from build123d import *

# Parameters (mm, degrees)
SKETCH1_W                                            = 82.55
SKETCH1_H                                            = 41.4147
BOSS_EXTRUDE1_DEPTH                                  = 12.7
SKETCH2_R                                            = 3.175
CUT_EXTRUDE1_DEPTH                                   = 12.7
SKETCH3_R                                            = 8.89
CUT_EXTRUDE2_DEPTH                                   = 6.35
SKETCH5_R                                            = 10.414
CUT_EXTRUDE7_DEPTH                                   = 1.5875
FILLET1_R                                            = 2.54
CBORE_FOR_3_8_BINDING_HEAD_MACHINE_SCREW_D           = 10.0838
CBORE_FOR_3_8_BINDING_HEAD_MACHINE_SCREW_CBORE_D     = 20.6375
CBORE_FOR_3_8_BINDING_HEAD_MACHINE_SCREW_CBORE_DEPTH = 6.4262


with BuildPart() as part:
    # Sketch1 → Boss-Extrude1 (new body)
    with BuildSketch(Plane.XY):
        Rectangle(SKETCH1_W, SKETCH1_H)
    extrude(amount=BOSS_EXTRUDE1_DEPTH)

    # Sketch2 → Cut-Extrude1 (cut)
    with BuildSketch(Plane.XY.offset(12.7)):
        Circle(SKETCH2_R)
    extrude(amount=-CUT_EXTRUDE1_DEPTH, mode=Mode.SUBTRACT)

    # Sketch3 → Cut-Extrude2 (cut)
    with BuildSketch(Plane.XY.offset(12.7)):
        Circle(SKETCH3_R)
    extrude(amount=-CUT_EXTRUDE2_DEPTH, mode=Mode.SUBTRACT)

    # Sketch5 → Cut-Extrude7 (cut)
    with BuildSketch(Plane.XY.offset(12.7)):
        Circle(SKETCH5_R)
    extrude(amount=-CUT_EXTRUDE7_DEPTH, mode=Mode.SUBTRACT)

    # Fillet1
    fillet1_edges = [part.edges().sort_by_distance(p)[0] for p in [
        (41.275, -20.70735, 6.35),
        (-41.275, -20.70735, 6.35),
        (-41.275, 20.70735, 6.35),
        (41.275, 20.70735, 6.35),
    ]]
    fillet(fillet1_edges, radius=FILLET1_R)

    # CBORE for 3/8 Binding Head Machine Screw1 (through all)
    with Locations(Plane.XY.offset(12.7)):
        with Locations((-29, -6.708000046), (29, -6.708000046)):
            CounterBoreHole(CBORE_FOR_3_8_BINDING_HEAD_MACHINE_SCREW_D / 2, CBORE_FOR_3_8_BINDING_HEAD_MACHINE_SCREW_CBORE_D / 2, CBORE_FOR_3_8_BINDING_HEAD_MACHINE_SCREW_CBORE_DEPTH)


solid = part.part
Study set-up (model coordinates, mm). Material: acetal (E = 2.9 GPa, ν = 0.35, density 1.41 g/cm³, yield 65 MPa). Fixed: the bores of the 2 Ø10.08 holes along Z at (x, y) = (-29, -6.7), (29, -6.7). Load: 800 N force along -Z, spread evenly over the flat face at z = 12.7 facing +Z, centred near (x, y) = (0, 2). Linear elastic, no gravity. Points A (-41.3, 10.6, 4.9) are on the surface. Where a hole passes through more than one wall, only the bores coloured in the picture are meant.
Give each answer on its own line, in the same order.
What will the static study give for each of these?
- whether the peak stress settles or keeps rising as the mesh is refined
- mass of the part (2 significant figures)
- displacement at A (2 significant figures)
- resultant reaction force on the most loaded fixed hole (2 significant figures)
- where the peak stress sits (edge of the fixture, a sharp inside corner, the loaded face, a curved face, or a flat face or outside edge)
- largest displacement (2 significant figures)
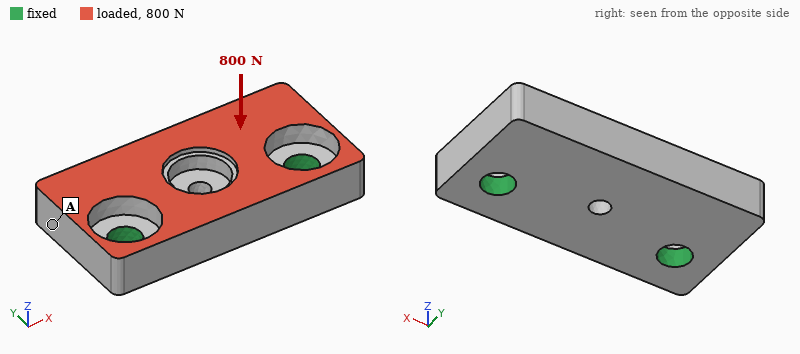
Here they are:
keeps rising
51 g
0.070 mm
410 N
edge of the fixture
0.20 mm
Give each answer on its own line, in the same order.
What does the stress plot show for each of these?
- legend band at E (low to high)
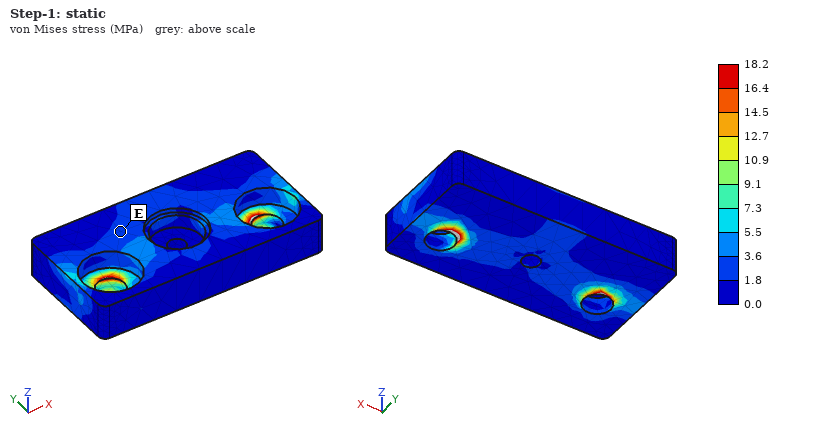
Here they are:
1.8 to 3.6 MPa
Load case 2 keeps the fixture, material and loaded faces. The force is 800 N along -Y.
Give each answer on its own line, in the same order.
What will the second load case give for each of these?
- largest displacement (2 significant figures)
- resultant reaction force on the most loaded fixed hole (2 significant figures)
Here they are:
0.19 mm
400 N
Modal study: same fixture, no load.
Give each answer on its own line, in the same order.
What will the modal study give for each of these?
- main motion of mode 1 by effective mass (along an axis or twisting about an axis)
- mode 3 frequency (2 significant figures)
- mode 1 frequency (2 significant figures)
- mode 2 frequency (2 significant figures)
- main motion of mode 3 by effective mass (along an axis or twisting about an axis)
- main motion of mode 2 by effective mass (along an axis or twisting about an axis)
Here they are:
along Z
3400 Hz
1700 Hz
3000 Hz
along Z
twisting about Y
